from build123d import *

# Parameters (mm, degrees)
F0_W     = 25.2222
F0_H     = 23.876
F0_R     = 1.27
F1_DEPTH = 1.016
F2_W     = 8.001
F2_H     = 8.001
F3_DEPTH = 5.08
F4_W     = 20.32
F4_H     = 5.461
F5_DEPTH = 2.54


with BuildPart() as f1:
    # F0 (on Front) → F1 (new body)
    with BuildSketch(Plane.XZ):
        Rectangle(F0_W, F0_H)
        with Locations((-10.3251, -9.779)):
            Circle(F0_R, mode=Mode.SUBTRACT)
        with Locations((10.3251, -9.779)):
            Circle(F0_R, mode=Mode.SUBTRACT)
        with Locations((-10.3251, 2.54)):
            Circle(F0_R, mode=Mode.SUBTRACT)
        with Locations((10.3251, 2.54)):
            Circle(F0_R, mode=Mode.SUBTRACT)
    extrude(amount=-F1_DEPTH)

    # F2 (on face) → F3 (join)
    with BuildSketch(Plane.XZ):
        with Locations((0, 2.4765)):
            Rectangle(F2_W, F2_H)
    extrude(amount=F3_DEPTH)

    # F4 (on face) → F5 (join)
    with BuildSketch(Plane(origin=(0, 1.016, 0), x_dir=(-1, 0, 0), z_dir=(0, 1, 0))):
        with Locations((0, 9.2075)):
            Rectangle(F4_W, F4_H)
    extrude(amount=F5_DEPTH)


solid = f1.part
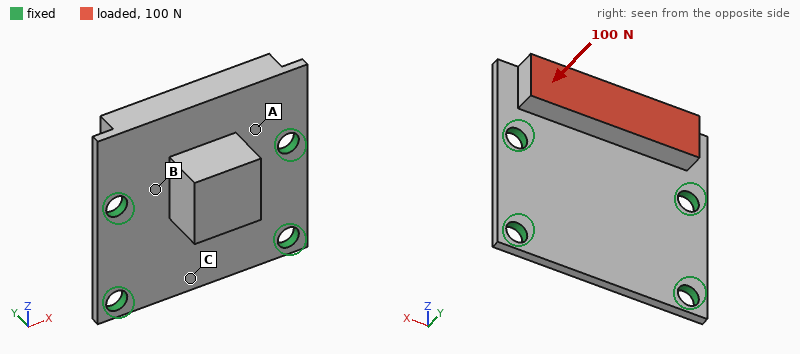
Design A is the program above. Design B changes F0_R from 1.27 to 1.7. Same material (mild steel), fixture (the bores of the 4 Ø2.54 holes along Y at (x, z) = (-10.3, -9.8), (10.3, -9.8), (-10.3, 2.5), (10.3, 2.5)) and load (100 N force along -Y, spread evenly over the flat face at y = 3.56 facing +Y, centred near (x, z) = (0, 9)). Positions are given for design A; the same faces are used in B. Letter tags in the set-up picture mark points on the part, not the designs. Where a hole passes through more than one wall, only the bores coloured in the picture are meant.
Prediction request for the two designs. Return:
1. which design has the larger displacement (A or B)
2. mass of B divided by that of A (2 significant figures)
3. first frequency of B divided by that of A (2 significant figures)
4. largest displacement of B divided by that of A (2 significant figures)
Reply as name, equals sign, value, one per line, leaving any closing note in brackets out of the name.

which design has the larger displacement = A
mass of B divided by that of A = 0.99
first frequency of B divided by that of A = 1.1
largest displacement of B divided by that of A = 0.82
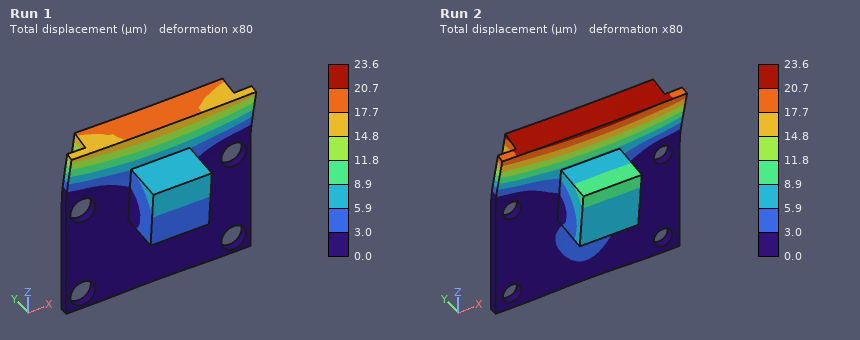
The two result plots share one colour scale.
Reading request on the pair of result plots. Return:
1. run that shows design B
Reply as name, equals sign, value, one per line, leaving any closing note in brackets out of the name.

run that shows design B = Run 1
